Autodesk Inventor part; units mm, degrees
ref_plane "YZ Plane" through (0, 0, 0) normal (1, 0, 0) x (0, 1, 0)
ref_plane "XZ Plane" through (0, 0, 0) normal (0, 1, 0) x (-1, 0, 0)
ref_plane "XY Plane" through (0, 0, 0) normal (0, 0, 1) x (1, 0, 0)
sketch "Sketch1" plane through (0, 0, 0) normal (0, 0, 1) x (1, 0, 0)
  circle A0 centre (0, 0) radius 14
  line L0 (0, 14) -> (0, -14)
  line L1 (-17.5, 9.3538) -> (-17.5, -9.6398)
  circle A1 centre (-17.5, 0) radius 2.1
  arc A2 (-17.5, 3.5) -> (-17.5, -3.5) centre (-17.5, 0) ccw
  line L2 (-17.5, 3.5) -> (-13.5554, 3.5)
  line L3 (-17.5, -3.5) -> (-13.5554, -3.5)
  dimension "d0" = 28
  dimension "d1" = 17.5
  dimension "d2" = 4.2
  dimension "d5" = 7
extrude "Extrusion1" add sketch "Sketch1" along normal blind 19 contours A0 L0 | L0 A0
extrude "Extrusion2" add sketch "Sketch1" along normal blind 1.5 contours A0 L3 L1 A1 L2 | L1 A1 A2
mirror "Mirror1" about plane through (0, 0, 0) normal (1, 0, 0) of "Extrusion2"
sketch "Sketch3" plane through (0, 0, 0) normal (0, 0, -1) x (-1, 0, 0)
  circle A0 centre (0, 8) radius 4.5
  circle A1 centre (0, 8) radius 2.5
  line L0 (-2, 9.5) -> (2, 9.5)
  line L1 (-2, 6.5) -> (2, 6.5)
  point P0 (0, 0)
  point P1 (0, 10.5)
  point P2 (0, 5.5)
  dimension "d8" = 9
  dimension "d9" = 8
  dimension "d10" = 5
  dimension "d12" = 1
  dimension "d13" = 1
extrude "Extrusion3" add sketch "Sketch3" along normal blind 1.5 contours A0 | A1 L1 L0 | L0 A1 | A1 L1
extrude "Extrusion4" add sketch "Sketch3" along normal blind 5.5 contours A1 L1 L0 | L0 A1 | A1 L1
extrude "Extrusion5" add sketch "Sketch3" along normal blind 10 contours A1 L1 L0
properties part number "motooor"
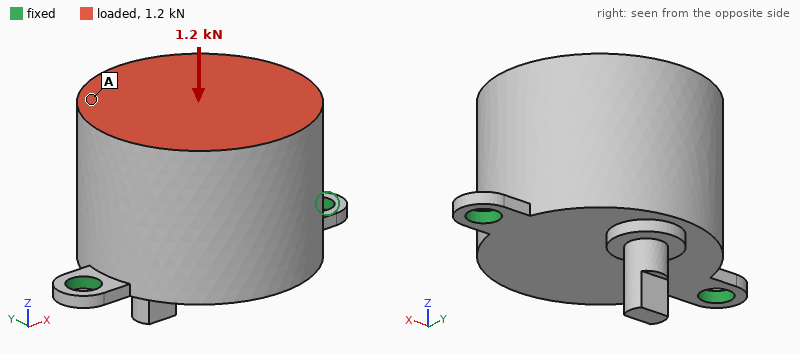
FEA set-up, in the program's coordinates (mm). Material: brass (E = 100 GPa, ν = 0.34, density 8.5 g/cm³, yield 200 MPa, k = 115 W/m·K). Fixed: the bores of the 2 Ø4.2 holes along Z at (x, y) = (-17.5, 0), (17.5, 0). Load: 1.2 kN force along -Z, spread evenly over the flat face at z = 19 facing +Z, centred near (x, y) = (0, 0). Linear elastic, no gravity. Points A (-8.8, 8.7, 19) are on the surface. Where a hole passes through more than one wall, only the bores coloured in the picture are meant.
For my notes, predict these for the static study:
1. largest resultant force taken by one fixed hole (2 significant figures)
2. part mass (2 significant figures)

690 N
100 g
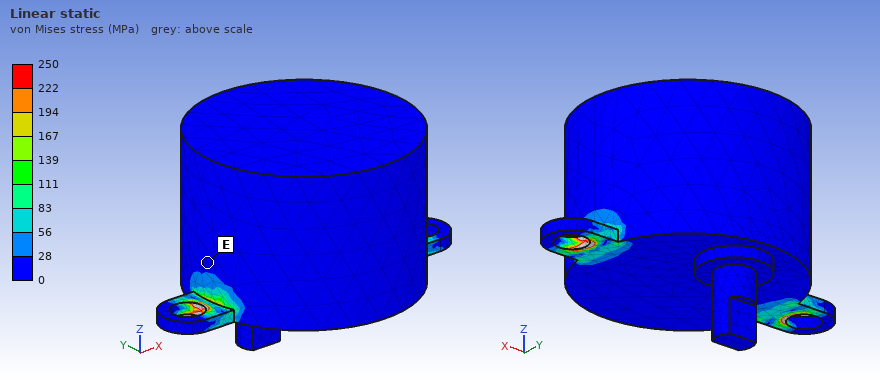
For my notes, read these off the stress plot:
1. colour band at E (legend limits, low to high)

0 to 28 MPa
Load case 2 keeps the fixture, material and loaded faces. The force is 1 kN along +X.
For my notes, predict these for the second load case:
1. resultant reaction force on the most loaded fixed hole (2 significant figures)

800 N
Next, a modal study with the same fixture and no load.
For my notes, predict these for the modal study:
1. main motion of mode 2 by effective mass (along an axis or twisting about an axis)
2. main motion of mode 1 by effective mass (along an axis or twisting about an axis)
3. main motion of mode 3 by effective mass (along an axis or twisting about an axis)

along Z
along Y
along X
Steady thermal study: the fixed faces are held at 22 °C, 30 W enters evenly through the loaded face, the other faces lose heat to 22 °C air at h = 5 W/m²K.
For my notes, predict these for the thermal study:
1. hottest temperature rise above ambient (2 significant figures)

54 K
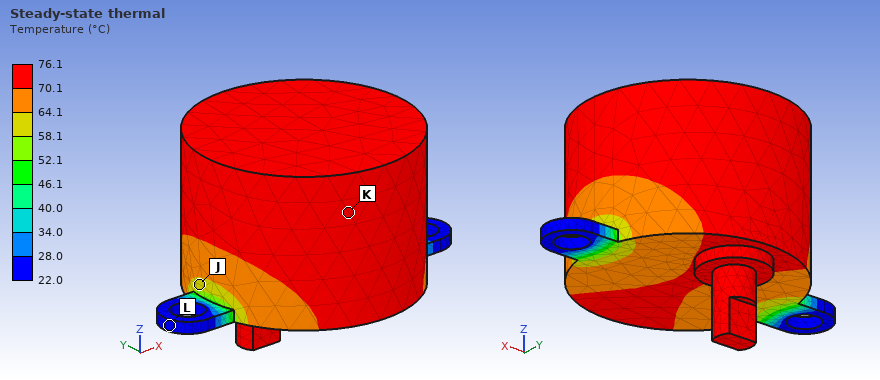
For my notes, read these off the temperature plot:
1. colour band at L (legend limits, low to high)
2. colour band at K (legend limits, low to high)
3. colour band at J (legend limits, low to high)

22.0 to 28.0 °C
70.1 to 76.1 °C
58.1 to 64.1 °C
